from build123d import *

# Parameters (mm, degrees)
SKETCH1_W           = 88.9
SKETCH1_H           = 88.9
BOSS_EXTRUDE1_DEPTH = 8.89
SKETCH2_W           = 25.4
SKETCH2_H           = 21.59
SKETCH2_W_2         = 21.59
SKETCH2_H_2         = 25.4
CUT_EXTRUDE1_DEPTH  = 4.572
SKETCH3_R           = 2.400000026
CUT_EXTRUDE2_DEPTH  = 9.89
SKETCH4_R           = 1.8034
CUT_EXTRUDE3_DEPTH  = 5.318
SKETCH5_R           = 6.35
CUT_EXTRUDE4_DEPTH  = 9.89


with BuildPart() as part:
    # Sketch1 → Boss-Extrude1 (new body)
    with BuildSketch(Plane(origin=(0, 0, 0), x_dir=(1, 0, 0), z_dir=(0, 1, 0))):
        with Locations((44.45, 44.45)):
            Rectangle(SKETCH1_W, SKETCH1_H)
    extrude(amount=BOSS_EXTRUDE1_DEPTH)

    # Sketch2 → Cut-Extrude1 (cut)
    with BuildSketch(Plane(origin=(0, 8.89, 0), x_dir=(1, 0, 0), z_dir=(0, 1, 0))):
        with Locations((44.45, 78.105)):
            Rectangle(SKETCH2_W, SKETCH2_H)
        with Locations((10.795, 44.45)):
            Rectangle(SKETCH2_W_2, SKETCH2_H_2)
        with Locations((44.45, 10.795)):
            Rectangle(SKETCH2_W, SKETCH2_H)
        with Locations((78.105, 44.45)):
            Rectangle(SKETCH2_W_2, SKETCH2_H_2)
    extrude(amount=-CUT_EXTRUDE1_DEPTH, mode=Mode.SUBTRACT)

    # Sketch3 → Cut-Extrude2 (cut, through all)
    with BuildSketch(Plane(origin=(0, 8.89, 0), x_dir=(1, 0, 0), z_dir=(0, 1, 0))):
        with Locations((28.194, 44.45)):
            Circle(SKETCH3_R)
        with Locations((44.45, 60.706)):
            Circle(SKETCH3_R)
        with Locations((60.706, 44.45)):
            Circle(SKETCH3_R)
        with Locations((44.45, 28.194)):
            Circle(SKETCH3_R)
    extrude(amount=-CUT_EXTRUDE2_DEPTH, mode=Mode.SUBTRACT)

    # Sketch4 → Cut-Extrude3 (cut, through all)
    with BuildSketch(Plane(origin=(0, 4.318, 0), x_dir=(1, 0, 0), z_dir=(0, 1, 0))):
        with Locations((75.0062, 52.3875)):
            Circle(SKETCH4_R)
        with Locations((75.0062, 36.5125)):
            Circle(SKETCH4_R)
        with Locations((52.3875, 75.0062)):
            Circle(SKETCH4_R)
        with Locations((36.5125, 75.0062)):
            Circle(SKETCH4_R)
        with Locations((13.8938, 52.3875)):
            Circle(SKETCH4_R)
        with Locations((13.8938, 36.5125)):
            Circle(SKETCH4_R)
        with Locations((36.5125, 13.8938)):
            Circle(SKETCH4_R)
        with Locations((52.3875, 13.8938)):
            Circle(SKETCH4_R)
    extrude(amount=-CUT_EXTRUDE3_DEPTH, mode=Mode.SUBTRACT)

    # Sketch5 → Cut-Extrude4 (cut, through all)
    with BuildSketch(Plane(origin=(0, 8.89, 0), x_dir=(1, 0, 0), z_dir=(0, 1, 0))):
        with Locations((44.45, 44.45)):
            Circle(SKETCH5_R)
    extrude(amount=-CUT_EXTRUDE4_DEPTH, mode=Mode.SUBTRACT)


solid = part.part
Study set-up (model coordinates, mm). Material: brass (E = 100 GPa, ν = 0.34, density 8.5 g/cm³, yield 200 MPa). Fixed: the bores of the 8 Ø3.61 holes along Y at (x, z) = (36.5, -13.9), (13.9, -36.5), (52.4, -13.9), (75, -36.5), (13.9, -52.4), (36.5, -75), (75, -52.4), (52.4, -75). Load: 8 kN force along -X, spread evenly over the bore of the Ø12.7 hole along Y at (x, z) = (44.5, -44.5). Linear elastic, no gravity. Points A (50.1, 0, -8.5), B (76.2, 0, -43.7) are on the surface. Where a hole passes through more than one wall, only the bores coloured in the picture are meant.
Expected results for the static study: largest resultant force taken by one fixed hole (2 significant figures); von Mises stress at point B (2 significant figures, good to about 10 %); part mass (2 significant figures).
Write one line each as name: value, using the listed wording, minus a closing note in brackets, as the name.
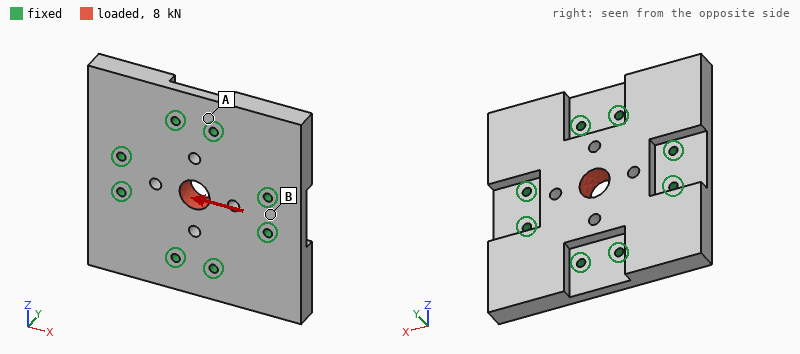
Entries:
largest resultant force taken by one fixed hole: 1.4 kN
von Mises stress at point B: 8.8 MPa
part mass: 490 g
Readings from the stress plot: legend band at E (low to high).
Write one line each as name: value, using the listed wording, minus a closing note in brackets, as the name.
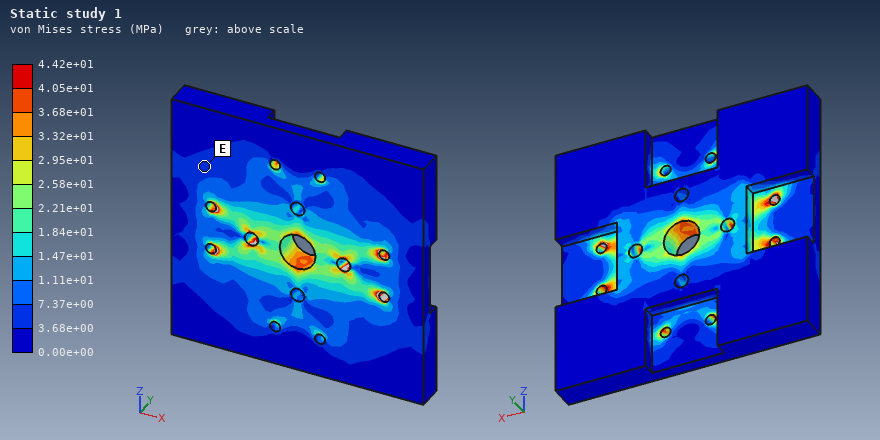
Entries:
legend band at E: 3.68e+00 to 7.37e+00 MPa
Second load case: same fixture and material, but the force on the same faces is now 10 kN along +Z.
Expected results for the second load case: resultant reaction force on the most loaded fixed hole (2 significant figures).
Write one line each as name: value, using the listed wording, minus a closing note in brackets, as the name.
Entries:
resultant reaction force on the most loaded fixed hole: 1.8 kN
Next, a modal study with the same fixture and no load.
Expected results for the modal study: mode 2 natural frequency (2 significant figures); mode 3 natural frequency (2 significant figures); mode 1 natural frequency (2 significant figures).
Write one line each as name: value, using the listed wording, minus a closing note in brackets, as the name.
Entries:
mode 2 natural frequency: 3700 Hz
mode 3 natural frequency: 3800 Hz
mode 1 natural frequency: 3600 Hz
